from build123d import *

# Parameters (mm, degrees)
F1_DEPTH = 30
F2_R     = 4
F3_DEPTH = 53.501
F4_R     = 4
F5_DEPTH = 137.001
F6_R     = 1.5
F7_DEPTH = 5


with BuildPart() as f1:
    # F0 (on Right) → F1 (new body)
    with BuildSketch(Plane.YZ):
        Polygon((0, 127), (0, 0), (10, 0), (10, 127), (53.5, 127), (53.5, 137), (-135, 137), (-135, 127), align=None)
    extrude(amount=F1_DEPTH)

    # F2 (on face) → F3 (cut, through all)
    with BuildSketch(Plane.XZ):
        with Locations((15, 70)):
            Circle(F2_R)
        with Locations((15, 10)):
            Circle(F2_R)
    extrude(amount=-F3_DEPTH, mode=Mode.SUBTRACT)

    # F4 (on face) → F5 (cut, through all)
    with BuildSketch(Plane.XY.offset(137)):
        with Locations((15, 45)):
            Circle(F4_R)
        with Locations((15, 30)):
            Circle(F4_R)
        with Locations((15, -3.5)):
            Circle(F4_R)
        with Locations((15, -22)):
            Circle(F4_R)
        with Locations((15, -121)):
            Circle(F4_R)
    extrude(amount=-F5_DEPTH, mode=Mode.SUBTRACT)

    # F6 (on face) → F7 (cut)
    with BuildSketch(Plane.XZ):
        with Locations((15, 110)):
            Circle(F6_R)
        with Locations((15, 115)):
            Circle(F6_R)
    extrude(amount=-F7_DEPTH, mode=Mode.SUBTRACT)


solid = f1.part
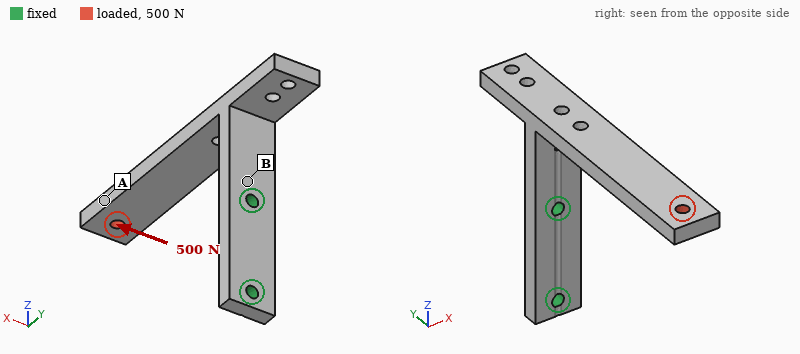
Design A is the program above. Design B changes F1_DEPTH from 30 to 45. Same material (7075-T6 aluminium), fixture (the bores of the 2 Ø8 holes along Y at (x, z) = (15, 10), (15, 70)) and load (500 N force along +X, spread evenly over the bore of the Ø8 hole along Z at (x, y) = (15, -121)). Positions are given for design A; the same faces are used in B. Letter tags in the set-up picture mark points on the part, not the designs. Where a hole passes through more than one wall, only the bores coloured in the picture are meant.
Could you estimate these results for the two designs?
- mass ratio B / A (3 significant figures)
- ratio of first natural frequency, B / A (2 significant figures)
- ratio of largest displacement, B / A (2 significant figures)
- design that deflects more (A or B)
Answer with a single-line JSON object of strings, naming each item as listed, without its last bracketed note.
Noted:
{"mass ratio B / A": "1.52", "ratio of first natural frequency, B / A": "1.00", "ratio of largest displacement, B / A": "0.59", "design that deflects more": "A"}
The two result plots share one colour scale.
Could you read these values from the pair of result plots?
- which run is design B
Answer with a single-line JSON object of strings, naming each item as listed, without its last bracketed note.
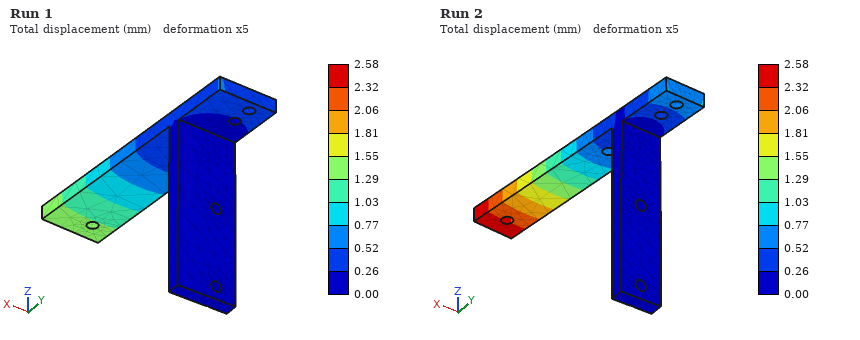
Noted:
{"which run is design B": "Run 1"}
